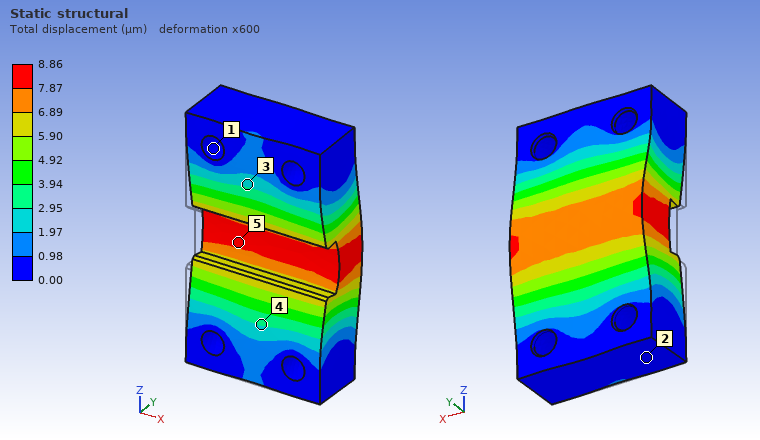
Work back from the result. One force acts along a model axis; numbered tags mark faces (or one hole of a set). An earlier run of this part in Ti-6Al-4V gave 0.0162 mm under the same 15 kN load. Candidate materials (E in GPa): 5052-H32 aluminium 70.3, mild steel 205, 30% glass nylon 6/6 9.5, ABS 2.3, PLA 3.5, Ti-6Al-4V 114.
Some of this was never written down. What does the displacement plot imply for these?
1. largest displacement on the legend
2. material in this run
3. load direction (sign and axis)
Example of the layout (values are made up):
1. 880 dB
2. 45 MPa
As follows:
1. 8.86 µm
2. mild steel
3. +Y
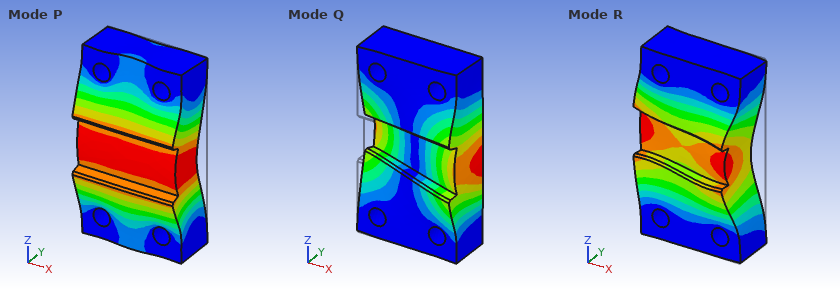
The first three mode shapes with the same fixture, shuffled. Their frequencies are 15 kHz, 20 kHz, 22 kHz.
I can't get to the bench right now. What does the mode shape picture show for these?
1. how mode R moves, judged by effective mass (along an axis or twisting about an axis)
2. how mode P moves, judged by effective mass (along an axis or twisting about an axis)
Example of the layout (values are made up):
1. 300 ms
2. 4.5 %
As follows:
1. along X
2. along Y
